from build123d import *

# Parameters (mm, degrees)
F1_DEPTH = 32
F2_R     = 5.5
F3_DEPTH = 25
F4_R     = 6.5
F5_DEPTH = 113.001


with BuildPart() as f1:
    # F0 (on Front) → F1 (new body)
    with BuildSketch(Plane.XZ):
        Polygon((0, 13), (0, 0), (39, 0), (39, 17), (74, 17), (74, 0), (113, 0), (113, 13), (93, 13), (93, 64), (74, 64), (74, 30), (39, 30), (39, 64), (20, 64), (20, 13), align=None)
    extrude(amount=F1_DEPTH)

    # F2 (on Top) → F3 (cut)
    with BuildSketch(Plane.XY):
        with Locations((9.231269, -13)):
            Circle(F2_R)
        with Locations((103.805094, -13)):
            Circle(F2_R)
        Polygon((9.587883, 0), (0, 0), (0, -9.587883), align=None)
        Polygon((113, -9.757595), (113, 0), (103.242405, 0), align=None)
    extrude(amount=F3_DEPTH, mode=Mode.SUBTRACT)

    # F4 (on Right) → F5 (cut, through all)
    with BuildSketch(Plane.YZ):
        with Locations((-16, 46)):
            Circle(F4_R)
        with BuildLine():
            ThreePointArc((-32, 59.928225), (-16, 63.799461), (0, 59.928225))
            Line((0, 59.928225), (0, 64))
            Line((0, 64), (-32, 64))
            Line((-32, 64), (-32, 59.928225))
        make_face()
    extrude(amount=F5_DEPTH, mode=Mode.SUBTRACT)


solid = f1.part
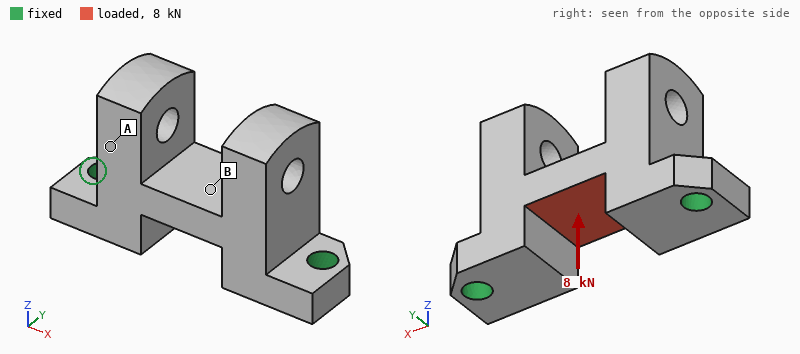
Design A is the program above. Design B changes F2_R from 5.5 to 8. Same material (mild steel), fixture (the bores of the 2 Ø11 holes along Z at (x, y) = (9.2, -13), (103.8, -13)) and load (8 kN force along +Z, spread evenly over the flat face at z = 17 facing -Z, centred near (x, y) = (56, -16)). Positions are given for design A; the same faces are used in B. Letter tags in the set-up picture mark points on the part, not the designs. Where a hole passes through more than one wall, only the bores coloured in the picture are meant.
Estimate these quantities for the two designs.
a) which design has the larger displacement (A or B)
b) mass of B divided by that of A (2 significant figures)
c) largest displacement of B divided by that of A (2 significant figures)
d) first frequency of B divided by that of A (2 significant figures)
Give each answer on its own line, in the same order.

A
0.97
0.84
1.2
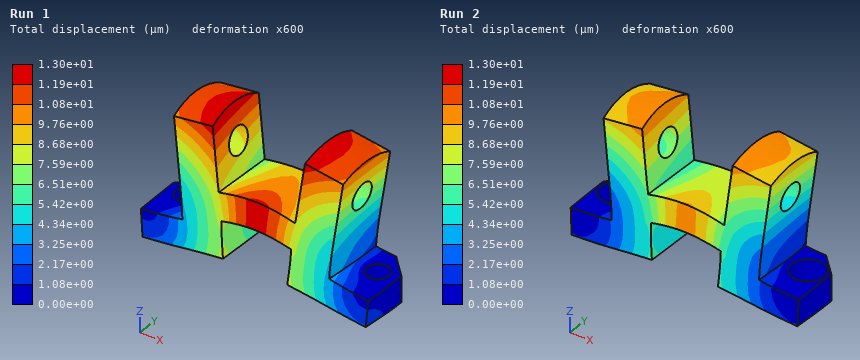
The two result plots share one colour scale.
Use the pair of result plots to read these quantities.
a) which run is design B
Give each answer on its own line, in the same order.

Run 2
